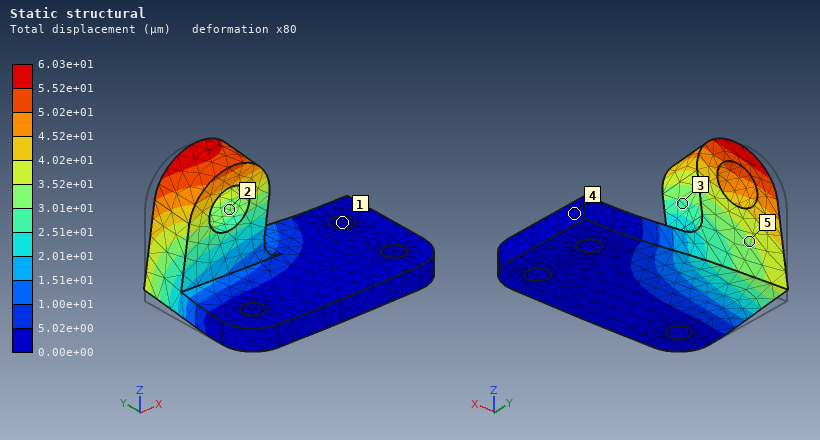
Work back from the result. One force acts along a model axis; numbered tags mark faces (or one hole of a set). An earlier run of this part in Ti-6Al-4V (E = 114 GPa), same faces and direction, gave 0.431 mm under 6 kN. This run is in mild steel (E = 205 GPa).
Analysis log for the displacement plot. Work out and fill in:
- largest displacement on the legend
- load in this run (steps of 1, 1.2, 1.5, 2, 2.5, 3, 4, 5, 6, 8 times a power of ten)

6.03e+01 µm
1.5 kN
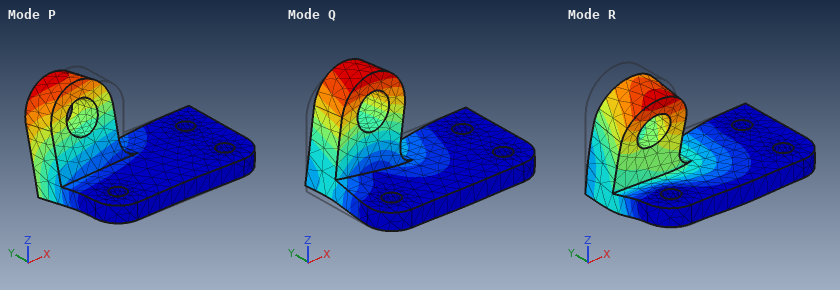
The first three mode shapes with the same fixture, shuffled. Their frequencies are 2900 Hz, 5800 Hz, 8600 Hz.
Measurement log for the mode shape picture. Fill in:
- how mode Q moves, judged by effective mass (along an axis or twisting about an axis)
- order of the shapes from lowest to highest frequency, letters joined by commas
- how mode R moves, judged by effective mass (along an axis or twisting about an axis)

along X
P, Q, R
along Z
